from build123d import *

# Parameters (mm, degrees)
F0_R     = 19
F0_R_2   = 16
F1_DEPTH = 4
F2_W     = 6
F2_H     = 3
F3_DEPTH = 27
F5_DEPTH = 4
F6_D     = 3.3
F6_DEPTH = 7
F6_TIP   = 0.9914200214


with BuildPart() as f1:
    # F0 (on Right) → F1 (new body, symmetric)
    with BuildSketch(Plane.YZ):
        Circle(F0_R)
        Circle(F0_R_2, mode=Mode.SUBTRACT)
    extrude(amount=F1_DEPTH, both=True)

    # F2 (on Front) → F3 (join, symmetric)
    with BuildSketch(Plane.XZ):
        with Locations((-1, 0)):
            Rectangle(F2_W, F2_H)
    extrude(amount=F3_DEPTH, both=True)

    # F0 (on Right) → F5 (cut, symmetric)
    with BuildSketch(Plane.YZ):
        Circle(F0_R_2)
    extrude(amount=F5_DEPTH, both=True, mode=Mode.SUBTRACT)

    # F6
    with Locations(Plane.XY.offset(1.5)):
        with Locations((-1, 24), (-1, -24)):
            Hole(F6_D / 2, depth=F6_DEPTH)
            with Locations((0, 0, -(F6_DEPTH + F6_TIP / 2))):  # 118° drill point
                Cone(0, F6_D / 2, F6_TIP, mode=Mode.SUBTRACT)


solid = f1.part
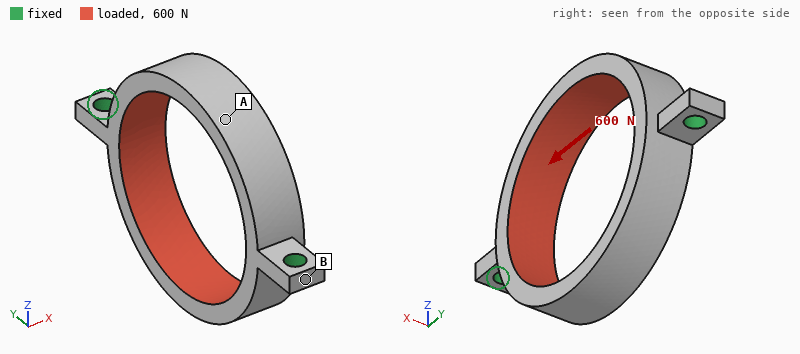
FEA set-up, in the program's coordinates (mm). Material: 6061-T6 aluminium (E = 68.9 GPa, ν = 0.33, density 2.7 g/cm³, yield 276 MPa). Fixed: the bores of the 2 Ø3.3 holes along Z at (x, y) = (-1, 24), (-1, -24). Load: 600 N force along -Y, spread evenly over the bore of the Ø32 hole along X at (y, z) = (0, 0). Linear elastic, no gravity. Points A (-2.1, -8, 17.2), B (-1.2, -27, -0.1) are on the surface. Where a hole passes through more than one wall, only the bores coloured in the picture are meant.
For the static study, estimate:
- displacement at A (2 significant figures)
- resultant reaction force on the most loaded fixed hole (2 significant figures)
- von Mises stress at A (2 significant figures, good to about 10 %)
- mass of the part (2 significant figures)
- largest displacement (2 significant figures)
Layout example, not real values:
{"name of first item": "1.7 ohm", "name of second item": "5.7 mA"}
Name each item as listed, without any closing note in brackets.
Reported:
{"displacement at A": "23 µm", "resultant reaction force on the most loaded fixed hole": "300 N", "von Mises stress at A": "21 MPa", "mass of the part": "7.8 g", "largest displacement": "25 µm"}
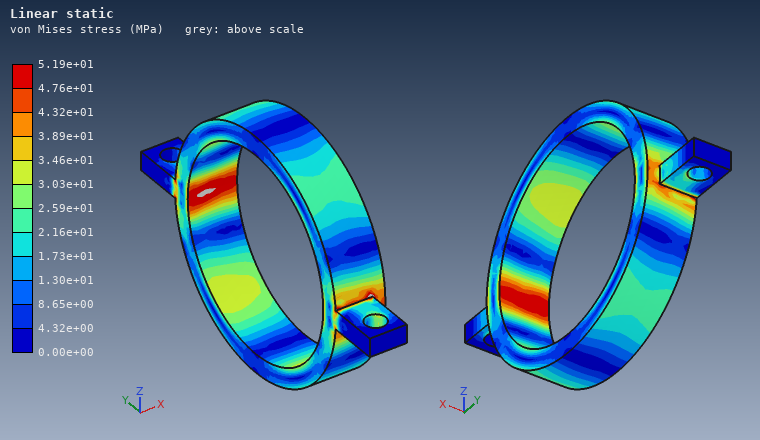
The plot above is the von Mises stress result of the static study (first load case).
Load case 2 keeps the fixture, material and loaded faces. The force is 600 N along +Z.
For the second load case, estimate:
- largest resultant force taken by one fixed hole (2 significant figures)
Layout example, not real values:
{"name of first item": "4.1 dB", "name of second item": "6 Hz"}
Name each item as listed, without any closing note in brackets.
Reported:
{"largest resultant force taken by one fixed hole": "300 N"}
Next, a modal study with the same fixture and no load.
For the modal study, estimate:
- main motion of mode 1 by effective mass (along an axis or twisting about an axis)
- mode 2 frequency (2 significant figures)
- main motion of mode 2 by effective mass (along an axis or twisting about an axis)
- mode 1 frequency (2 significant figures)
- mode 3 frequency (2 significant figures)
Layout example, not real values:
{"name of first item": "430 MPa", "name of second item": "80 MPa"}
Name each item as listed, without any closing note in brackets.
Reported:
{"main motion of mode 1 by effective mass": "twisting about Y", "mode 2 frequency": "6700 Hz", "main motion of mode 2 by effective mass": "along X", "mode 1 frequency": "3300 Hz", "mode 3 frequency": "7000 Hz"}
